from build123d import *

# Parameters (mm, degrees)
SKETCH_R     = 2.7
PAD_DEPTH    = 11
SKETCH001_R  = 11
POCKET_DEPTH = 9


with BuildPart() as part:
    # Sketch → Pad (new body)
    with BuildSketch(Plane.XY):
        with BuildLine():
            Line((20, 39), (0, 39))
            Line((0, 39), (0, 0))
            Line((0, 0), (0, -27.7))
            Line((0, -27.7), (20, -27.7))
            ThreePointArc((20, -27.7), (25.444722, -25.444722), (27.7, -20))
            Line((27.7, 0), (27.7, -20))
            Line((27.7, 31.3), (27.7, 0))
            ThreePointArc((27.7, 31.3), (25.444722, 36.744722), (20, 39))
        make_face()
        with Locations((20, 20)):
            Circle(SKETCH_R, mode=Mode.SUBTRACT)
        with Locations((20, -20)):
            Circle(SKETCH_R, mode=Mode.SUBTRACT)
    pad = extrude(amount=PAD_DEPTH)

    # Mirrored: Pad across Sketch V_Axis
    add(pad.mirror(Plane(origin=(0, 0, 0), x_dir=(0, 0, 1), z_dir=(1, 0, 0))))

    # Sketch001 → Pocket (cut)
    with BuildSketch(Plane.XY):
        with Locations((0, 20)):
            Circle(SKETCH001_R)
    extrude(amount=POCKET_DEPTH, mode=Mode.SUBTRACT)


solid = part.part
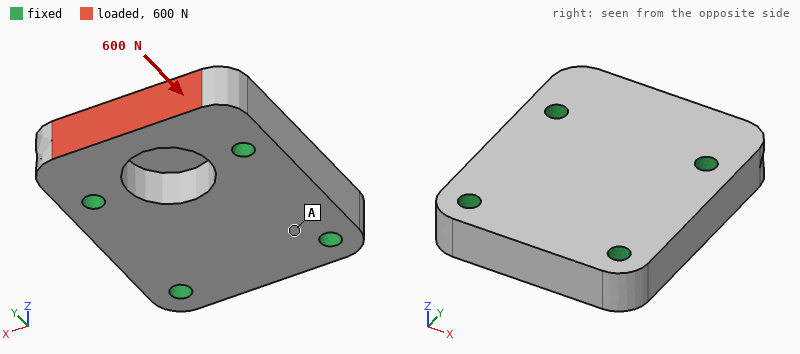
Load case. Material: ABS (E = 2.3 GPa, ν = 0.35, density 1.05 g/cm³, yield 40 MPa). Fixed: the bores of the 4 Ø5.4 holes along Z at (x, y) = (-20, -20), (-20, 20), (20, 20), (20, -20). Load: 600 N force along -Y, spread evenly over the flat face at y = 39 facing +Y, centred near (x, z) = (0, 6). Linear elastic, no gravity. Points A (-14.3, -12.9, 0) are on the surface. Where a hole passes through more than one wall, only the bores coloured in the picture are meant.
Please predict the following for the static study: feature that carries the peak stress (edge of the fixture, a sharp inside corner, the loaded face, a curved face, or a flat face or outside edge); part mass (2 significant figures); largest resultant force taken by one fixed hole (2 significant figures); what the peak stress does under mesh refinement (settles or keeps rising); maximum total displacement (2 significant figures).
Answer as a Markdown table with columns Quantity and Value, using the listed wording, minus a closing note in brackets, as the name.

| Quantity | Value |
|---|---|
| feature that carries the peak stress | edge of the fixture |
| part mass | 37 g |
| largest resultant force taken by one fixed hole | 290 N |
| what the peak stress does under mesh refinement | keeps rising |
| maximum total displacement | 37 µm |
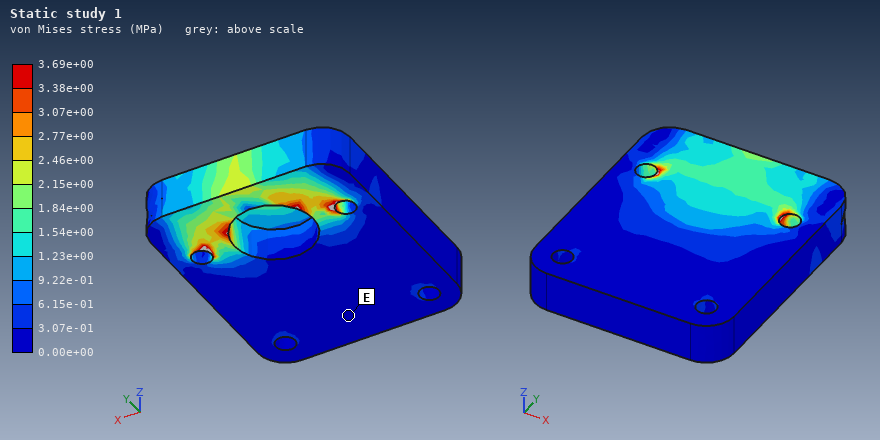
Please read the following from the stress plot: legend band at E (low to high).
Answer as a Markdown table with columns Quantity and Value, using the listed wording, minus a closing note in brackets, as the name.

| Quantity | Value |
|---|---|
| legend band at E | 0.00e+00 to 3.07e-01 MPa |
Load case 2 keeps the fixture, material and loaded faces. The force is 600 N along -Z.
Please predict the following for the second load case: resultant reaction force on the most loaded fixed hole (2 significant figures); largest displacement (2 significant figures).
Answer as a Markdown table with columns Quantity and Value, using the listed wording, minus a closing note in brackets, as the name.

| Quantity | Value |
|---|---|
| resultant reaction force on the most loaded fixed hole | 340 N |
| largest displacement | 0.28 mm |
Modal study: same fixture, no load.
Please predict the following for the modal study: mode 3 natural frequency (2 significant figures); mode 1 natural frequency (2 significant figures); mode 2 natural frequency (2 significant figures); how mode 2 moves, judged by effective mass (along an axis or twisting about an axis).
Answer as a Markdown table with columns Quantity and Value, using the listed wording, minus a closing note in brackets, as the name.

| Quantity | Value |
|---|---|
| mode 3 natural frequency | 7200 Hz |
| mode 1 natural frequency | 4700 Hz |
| mode 2 natural frequency | 5700 Hz |
| how mode 2 moves, judged by effective mass | along Z |
